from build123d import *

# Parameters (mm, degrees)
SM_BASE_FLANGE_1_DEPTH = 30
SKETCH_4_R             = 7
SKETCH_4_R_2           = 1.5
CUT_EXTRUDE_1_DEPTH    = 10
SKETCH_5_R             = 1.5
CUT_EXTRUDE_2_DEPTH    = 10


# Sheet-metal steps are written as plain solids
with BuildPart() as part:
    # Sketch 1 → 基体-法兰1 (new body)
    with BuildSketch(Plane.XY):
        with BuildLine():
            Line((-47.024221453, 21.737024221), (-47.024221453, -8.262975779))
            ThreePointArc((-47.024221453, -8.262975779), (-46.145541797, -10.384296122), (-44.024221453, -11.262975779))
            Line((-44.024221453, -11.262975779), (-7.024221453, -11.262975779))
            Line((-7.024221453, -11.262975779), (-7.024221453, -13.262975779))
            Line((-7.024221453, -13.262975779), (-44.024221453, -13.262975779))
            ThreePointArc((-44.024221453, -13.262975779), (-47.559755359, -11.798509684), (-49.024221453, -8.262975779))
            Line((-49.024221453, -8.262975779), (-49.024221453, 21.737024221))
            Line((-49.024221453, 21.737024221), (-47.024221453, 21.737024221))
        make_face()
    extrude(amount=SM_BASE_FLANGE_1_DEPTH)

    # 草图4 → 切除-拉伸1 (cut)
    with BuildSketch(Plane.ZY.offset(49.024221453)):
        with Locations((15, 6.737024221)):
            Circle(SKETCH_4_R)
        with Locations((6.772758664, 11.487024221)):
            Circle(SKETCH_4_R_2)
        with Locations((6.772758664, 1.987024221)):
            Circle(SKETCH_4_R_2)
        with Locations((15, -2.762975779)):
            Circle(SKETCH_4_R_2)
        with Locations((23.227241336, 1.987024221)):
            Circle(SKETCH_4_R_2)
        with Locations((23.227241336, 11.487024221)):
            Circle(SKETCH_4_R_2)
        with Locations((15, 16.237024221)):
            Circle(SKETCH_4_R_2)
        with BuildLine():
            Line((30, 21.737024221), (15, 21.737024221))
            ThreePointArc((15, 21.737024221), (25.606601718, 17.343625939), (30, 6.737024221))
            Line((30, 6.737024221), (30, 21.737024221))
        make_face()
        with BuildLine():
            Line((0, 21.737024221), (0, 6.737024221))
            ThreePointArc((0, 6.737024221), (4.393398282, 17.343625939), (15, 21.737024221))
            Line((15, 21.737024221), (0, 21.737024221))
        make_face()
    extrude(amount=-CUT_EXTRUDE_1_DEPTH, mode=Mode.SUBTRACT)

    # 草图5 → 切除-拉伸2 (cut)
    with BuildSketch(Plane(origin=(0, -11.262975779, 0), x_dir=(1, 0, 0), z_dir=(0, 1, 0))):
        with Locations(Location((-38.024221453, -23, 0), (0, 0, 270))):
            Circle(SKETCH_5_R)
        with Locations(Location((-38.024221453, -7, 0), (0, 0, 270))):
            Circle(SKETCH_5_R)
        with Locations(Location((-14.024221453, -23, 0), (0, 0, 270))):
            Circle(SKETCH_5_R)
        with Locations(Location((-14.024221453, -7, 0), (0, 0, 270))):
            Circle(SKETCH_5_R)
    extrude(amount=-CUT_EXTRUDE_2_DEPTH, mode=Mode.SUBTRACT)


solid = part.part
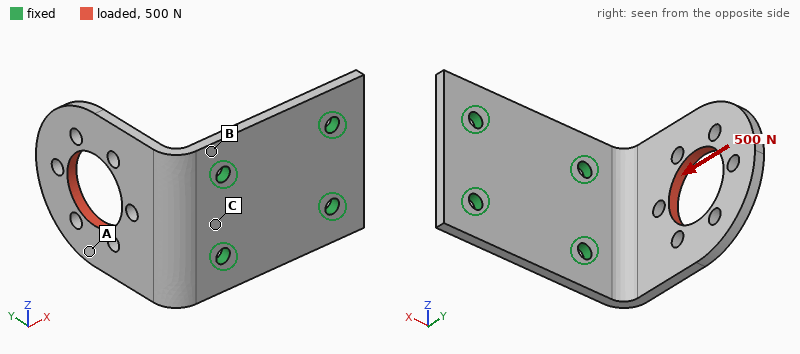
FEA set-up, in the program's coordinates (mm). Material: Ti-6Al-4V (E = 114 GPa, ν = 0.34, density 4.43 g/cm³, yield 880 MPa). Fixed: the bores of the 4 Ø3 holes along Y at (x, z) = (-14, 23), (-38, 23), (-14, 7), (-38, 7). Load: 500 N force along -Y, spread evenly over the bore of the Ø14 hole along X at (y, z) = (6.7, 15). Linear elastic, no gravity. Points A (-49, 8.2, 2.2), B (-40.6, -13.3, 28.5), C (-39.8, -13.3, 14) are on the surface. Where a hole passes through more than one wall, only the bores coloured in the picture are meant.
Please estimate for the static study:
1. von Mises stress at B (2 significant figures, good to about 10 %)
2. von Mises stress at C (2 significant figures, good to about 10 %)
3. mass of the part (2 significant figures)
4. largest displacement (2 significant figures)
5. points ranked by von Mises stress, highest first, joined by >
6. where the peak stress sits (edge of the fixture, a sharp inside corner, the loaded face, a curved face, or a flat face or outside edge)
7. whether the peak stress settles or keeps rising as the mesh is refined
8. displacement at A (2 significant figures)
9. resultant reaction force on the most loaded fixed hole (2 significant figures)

130 MPa
100 MPa
17 g
0.35 mm
B > C > A
edge of the fixture
keeps rising
0.22 mm
260 N
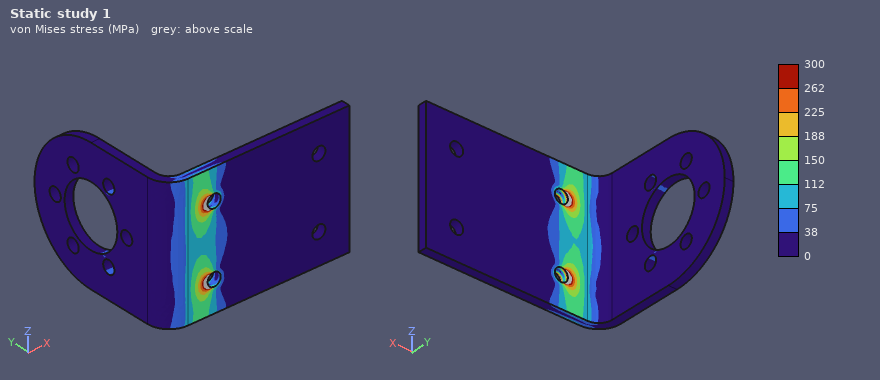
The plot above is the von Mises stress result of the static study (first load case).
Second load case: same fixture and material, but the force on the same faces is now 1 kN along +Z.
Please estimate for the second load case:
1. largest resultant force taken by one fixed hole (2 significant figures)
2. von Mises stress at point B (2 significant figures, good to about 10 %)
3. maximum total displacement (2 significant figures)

1.2 kN
350 MPa
0.55 mm
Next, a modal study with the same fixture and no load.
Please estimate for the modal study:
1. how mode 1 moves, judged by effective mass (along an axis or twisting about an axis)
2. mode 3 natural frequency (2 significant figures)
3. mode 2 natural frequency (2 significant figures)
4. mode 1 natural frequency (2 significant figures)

along X
4700 Hz
3100 Hz
1300 Hz
